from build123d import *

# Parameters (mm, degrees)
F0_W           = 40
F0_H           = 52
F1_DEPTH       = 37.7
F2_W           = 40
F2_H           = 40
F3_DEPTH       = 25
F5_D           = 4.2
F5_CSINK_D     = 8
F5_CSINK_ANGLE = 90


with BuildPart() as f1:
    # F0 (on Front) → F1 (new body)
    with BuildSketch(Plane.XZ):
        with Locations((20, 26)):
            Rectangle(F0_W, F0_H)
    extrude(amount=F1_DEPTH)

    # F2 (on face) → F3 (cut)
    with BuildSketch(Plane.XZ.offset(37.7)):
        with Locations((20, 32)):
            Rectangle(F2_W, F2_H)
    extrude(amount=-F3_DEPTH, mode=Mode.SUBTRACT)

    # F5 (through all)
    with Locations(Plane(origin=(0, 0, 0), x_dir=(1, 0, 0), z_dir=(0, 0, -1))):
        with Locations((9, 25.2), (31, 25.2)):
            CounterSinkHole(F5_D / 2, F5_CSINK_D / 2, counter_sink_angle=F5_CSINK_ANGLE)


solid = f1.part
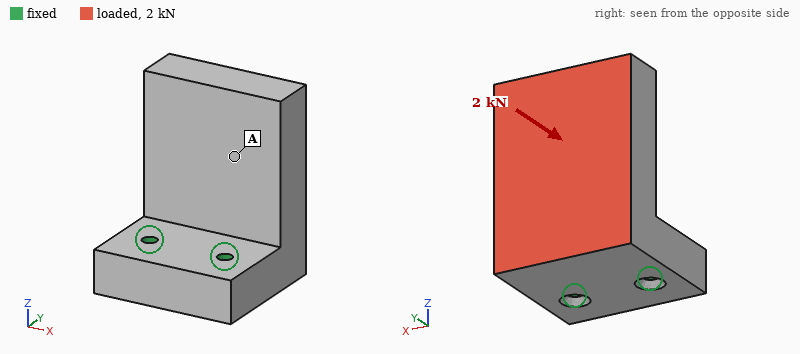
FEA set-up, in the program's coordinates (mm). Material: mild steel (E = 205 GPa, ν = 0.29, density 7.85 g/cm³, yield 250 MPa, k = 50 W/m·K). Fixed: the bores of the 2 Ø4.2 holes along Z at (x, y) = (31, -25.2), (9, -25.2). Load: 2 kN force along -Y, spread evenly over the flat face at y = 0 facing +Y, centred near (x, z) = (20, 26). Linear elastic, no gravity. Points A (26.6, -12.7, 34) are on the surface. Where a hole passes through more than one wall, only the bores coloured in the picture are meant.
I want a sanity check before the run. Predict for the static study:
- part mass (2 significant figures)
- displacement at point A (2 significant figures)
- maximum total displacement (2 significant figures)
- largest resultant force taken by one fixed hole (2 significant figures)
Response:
300 g
25 µm
46 µm
1.0 kN
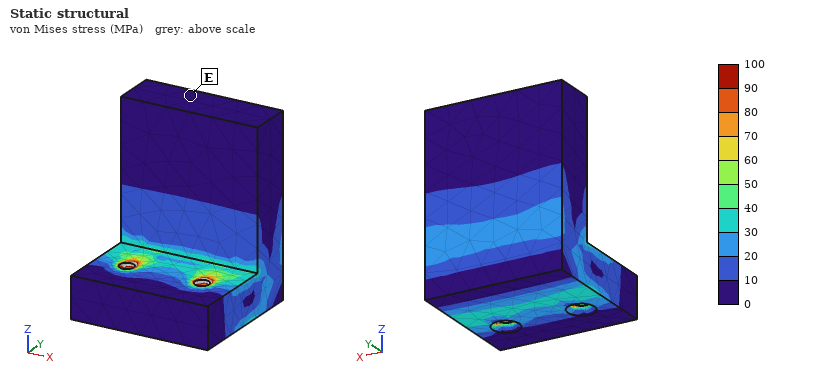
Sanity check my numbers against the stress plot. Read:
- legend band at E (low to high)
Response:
0 to 10 MPa
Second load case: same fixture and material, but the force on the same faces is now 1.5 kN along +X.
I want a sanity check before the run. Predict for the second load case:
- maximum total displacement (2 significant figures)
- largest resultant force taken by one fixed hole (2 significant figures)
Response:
12 µm
2.0 kN
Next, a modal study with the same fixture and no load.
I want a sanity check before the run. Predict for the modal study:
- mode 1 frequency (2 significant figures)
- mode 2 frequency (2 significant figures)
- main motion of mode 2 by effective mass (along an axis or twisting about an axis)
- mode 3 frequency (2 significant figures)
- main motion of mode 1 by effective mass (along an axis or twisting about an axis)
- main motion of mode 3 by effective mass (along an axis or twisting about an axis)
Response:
2700 Hz
4600 Hz
along X
8900 Hz
along Y
along Z
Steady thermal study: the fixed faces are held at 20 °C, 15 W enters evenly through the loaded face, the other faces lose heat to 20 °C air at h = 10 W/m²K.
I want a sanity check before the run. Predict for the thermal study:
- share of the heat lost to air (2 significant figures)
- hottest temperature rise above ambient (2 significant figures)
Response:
4.9 %
21 K
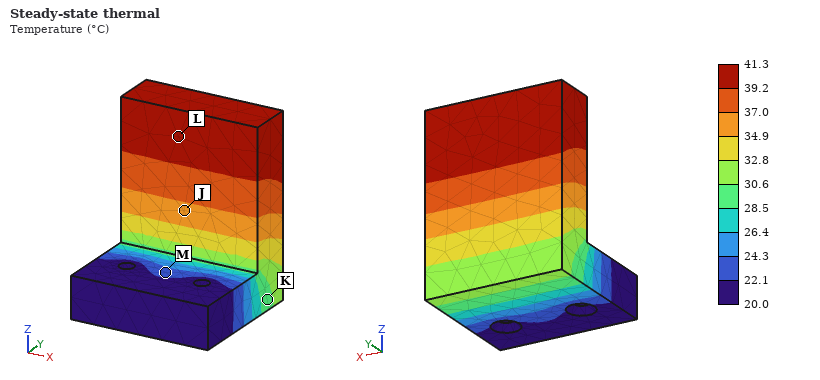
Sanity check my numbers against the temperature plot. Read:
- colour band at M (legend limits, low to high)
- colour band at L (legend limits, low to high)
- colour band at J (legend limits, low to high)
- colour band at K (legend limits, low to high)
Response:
22.1 to 24.3 °C
39.2 to 41.3 °C
34.9 to 37.0 °C
28.5 to 30.6 °C
